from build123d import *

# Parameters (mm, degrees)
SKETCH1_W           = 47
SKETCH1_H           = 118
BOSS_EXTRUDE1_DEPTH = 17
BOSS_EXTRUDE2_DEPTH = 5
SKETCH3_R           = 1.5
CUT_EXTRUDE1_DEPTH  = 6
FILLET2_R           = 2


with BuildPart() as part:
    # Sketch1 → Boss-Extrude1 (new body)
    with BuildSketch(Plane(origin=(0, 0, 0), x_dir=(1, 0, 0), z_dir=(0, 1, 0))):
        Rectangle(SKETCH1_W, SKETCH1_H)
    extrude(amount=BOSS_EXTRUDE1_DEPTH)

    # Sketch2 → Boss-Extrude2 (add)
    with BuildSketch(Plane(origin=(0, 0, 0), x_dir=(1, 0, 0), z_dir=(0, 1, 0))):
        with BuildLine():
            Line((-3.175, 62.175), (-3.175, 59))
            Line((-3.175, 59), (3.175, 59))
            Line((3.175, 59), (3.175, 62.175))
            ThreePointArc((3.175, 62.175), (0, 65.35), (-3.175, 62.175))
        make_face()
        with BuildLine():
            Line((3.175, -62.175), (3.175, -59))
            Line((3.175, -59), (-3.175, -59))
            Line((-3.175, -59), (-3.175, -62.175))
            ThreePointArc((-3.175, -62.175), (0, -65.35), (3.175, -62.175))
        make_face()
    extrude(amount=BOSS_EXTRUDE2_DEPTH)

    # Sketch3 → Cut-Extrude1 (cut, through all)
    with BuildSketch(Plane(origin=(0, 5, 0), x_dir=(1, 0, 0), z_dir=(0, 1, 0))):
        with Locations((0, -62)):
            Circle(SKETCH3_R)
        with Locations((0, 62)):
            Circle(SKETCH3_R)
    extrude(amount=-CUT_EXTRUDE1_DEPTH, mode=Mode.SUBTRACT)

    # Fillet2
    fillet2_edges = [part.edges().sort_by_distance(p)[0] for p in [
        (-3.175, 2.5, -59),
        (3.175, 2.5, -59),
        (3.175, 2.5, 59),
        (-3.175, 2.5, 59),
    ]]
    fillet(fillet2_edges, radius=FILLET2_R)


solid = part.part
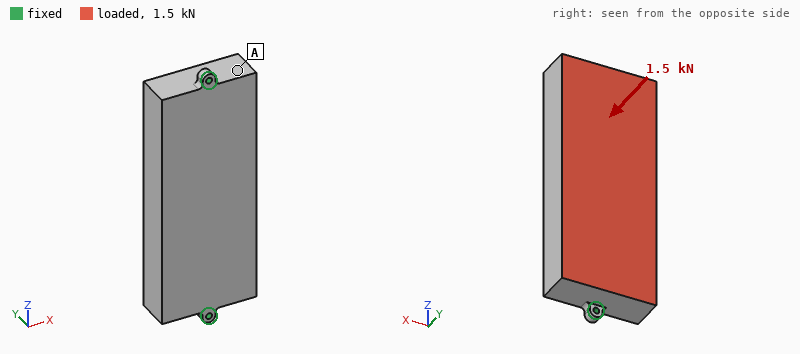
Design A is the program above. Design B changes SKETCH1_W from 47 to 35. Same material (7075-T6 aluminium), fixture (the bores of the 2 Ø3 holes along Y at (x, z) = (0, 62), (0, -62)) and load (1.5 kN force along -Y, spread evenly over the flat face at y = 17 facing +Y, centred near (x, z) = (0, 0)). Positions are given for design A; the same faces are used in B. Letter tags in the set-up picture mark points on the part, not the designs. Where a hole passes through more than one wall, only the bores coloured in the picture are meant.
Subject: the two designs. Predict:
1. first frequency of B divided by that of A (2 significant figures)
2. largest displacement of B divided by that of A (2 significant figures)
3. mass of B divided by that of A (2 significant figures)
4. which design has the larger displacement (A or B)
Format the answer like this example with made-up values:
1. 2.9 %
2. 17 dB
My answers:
1. 1.4
2. 1.2
3. 0.75
4. B
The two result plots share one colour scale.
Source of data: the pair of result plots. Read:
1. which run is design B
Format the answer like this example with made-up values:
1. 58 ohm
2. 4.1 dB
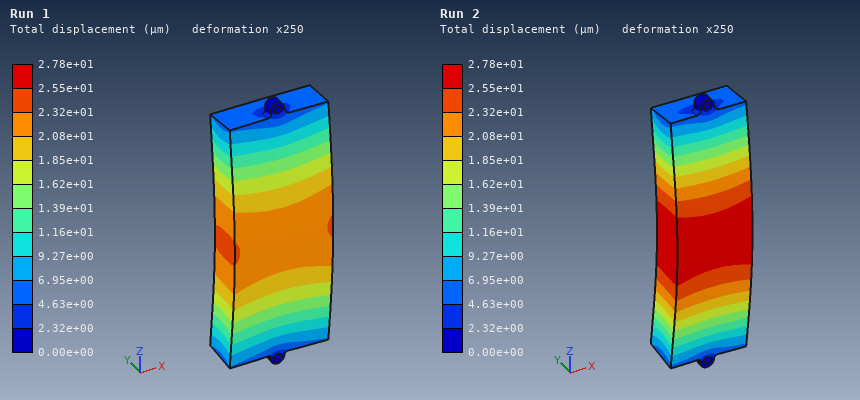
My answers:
1. Run 2
